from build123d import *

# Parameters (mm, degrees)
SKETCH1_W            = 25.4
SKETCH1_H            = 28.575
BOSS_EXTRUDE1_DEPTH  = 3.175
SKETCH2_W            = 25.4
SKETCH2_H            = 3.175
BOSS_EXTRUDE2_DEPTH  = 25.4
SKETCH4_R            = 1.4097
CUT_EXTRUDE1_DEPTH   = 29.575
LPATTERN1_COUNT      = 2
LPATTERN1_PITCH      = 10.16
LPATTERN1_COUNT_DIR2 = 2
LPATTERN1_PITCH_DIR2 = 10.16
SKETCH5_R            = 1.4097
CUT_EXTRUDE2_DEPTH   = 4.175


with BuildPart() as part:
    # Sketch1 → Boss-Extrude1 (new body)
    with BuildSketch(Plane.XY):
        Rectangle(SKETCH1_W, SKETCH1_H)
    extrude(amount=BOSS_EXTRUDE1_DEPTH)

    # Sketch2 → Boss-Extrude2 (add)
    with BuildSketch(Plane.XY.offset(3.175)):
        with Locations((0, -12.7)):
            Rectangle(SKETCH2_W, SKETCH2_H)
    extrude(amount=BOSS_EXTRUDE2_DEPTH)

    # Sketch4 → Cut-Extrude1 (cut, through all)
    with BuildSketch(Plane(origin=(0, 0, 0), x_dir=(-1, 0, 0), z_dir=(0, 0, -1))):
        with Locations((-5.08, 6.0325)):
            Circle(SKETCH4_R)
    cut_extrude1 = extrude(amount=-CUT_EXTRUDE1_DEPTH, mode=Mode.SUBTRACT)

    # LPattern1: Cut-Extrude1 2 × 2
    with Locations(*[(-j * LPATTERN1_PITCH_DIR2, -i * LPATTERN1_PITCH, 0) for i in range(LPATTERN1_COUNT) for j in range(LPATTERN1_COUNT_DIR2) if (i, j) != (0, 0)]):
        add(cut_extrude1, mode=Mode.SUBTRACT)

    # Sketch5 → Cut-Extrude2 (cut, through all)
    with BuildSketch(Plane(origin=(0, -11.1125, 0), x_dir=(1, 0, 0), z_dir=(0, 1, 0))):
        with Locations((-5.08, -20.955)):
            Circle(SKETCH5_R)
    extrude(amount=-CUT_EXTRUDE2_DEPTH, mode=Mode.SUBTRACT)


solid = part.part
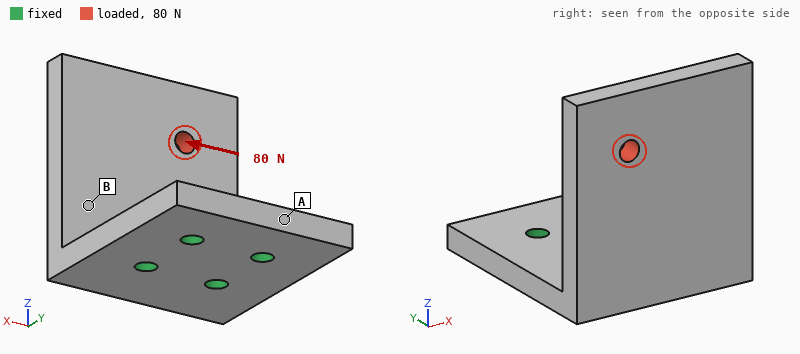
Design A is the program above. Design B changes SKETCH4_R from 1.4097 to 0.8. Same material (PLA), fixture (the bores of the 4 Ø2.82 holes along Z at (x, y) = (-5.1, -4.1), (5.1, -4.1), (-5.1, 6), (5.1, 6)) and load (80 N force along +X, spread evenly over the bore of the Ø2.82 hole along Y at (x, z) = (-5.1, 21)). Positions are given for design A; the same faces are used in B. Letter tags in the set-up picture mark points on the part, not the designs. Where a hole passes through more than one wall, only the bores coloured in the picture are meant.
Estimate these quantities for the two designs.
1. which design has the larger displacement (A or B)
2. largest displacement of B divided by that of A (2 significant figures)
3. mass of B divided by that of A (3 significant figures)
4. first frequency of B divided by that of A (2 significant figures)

B
1.2
1.01
0.96
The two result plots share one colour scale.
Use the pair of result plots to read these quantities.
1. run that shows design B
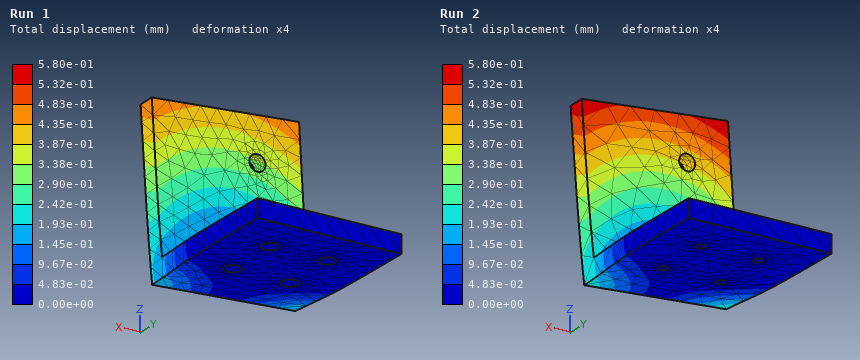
Run 2
